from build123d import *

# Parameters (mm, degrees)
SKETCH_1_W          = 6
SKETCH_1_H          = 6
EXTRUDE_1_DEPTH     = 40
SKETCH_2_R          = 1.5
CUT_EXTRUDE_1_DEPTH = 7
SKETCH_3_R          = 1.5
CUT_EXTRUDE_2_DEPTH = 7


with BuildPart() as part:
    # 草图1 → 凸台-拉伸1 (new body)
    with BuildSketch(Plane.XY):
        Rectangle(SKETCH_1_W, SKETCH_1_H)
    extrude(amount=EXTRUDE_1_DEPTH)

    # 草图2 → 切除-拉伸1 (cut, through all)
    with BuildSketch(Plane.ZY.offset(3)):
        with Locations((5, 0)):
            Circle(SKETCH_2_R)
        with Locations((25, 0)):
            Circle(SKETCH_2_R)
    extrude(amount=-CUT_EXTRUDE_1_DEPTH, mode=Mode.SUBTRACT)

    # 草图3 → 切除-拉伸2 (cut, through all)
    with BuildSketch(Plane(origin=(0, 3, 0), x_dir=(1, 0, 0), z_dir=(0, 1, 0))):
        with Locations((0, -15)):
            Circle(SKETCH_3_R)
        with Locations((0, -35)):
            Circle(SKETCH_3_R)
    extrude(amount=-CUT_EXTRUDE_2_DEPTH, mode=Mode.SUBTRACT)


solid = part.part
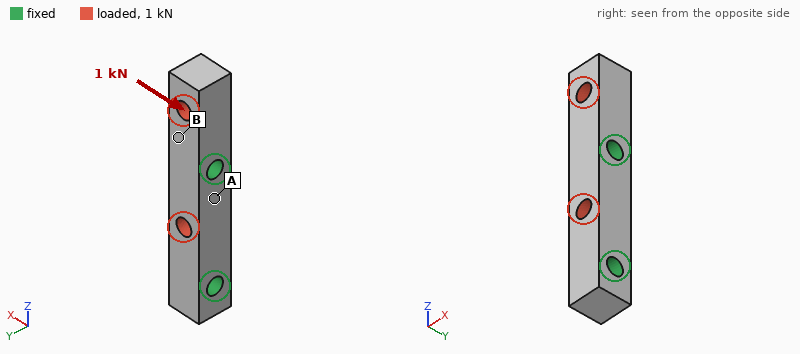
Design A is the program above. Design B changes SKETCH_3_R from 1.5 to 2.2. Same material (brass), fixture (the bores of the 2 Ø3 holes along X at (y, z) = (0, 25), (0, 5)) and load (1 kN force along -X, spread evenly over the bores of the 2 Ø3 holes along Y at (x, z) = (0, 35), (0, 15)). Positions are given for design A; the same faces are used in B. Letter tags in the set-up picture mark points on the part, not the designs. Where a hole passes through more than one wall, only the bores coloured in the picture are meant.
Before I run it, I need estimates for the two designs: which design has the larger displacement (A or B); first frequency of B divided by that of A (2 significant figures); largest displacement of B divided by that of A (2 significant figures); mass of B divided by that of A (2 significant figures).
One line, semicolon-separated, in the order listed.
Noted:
B; 1.00; 1.4; 0.92
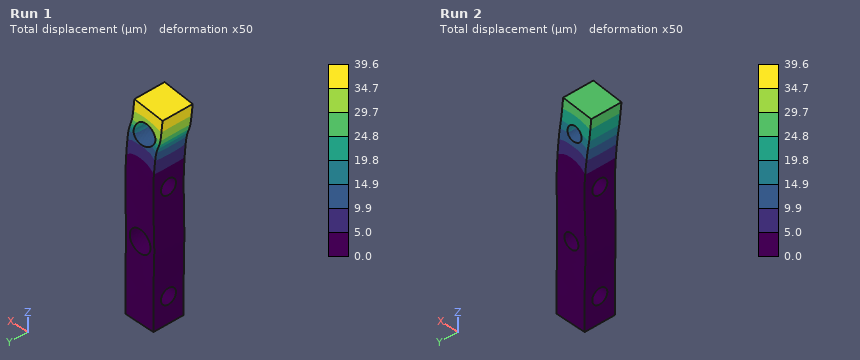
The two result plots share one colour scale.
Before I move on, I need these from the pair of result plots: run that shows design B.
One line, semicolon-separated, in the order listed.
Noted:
Run 1
